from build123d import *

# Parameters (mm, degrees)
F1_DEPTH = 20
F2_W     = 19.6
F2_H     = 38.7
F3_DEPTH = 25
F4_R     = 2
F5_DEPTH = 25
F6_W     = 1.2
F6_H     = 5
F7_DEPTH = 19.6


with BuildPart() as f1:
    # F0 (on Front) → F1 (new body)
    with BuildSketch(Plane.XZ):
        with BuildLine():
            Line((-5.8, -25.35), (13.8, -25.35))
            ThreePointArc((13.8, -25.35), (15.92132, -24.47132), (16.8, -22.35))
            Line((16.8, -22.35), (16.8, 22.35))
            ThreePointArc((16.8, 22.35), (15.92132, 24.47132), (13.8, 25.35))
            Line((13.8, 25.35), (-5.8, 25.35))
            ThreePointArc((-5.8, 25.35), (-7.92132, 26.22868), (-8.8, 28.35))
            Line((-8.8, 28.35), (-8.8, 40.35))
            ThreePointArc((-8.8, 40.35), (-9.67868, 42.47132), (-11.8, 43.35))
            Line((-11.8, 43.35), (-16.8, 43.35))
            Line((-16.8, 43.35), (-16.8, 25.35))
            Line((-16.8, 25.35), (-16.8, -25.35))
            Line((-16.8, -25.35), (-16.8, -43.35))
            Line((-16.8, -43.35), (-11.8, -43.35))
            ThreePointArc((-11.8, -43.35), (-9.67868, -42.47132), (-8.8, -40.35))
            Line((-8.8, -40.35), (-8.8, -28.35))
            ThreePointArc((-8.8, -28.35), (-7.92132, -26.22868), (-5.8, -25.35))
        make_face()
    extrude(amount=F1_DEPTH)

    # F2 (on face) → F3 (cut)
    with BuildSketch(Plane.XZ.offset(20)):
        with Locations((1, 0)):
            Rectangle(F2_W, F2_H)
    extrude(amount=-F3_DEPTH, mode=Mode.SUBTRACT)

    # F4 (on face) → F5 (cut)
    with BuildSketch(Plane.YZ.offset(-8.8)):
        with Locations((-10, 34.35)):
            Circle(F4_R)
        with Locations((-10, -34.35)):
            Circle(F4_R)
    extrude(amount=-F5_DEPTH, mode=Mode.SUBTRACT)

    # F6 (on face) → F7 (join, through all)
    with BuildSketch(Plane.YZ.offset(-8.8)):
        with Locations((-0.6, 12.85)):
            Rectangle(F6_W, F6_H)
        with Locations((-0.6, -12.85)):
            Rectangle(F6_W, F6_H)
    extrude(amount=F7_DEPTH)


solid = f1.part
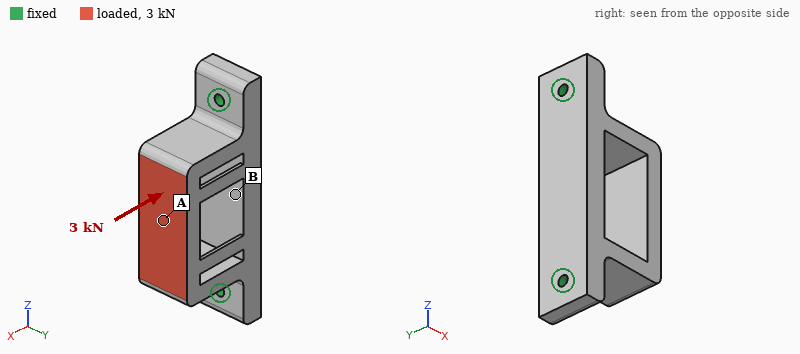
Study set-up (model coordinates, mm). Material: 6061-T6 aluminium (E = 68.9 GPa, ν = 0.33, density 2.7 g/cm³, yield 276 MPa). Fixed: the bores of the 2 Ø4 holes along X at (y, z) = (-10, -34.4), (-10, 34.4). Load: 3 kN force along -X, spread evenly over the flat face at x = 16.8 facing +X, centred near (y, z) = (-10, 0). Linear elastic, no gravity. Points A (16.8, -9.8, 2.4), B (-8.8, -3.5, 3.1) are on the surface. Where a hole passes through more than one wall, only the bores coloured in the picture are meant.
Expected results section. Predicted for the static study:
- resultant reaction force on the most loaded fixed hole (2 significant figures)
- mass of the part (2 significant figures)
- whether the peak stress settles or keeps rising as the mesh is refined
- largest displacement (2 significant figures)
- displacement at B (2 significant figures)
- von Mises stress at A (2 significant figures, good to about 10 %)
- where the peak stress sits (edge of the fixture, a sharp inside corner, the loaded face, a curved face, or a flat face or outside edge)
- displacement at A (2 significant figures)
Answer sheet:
1.6 kN
66 g
keeps rising
58 µm
20 µm
48 MPa
edge of the fixture
49 µm
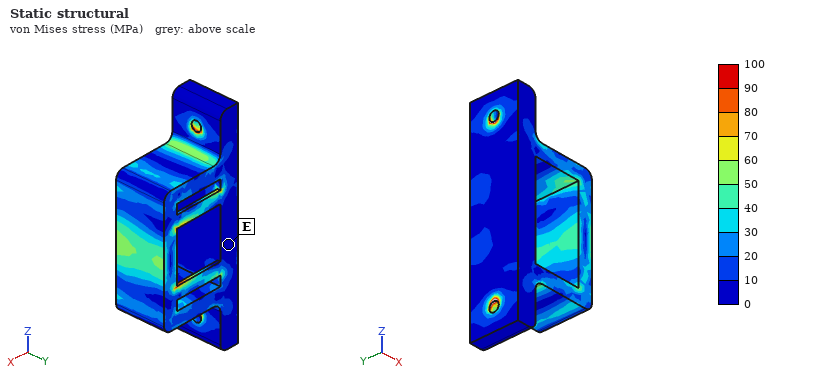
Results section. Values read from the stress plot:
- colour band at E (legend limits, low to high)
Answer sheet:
0 to 10 MPa
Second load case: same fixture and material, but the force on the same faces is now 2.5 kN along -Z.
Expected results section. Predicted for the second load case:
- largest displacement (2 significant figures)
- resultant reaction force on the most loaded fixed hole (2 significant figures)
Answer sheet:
0.10 mm
1.7 kN
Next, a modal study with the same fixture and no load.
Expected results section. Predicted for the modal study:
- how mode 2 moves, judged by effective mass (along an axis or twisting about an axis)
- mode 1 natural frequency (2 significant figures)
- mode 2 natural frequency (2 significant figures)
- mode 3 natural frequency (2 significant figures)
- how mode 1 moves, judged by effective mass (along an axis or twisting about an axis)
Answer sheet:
along Z
4000 Hz
5800 Hz
8000 Hz
along Y
